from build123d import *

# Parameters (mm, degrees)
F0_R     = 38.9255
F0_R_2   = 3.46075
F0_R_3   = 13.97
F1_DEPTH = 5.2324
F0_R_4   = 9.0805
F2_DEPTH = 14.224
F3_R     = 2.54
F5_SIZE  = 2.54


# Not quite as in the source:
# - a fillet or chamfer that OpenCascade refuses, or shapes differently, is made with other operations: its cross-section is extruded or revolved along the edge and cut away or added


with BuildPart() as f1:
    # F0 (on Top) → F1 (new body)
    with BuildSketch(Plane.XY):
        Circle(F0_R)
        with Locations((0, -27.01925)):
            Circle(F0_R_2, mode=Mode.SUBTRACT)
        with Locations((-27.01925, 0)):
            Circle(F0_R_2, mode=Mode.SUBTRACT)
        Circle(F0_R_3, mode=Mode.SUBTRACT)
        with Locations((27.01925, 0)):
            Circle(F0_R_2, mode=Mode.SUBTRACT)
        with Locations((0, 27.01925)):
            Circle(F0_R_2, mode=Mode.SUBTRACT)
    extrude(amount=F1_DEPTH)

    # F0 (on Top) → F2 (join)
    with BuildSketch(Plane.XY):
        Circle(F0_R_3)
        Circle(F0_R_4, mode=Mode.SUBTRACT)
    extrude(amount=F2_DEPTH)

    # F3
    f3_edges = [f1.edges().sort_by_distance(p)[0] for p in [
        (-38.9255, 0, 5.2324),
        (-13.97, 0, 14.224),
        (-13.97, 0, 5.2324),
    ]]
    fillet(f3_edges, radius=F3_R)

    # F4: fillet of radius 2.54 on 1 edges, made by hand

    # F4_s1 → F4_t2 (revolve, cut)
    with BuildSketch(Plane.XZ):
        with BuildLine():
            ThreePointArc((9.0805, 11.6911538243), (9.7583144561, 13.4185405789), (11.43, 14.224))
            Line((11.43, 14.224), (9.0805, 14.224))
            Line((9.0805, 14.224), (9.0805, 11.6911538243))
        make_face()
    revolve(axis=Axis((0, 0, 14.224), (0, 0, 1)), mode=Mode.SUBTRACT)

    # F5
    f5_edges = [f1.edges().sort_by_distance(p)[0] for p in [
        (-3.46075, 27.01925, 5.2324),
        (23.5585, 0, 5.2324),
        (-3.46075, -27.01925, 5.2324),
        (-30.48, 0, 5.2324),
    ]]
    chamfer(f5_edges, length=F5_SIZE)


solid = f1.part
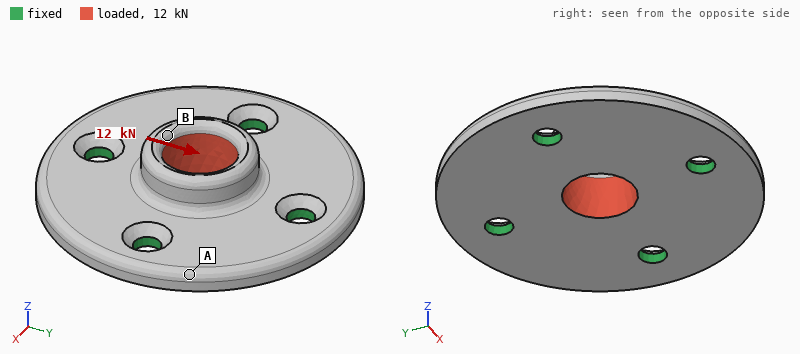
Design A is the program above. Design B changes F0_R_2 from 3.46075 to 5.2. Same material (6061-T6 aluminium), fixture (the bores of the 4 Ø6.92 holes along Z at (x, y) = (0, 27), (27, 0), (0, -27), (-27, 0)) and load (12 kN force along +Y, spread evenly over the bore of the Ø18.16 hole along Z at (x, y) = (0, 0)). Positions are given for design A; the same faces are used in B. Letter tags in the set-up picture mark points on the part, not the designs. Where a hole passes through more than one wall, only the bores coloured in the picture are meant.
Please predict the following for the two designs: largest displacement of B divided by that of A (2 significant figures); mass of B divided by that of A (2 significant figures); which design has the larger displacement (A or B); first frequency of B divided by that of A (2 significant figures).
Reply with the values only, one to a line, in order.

0.83
0.96
A
1.2
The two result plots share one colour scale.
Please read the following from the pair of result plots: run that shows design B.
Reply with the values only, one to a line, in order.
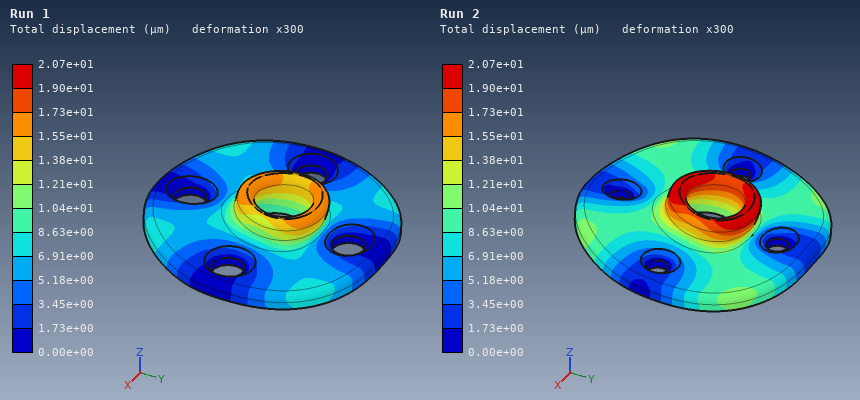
Run 1
